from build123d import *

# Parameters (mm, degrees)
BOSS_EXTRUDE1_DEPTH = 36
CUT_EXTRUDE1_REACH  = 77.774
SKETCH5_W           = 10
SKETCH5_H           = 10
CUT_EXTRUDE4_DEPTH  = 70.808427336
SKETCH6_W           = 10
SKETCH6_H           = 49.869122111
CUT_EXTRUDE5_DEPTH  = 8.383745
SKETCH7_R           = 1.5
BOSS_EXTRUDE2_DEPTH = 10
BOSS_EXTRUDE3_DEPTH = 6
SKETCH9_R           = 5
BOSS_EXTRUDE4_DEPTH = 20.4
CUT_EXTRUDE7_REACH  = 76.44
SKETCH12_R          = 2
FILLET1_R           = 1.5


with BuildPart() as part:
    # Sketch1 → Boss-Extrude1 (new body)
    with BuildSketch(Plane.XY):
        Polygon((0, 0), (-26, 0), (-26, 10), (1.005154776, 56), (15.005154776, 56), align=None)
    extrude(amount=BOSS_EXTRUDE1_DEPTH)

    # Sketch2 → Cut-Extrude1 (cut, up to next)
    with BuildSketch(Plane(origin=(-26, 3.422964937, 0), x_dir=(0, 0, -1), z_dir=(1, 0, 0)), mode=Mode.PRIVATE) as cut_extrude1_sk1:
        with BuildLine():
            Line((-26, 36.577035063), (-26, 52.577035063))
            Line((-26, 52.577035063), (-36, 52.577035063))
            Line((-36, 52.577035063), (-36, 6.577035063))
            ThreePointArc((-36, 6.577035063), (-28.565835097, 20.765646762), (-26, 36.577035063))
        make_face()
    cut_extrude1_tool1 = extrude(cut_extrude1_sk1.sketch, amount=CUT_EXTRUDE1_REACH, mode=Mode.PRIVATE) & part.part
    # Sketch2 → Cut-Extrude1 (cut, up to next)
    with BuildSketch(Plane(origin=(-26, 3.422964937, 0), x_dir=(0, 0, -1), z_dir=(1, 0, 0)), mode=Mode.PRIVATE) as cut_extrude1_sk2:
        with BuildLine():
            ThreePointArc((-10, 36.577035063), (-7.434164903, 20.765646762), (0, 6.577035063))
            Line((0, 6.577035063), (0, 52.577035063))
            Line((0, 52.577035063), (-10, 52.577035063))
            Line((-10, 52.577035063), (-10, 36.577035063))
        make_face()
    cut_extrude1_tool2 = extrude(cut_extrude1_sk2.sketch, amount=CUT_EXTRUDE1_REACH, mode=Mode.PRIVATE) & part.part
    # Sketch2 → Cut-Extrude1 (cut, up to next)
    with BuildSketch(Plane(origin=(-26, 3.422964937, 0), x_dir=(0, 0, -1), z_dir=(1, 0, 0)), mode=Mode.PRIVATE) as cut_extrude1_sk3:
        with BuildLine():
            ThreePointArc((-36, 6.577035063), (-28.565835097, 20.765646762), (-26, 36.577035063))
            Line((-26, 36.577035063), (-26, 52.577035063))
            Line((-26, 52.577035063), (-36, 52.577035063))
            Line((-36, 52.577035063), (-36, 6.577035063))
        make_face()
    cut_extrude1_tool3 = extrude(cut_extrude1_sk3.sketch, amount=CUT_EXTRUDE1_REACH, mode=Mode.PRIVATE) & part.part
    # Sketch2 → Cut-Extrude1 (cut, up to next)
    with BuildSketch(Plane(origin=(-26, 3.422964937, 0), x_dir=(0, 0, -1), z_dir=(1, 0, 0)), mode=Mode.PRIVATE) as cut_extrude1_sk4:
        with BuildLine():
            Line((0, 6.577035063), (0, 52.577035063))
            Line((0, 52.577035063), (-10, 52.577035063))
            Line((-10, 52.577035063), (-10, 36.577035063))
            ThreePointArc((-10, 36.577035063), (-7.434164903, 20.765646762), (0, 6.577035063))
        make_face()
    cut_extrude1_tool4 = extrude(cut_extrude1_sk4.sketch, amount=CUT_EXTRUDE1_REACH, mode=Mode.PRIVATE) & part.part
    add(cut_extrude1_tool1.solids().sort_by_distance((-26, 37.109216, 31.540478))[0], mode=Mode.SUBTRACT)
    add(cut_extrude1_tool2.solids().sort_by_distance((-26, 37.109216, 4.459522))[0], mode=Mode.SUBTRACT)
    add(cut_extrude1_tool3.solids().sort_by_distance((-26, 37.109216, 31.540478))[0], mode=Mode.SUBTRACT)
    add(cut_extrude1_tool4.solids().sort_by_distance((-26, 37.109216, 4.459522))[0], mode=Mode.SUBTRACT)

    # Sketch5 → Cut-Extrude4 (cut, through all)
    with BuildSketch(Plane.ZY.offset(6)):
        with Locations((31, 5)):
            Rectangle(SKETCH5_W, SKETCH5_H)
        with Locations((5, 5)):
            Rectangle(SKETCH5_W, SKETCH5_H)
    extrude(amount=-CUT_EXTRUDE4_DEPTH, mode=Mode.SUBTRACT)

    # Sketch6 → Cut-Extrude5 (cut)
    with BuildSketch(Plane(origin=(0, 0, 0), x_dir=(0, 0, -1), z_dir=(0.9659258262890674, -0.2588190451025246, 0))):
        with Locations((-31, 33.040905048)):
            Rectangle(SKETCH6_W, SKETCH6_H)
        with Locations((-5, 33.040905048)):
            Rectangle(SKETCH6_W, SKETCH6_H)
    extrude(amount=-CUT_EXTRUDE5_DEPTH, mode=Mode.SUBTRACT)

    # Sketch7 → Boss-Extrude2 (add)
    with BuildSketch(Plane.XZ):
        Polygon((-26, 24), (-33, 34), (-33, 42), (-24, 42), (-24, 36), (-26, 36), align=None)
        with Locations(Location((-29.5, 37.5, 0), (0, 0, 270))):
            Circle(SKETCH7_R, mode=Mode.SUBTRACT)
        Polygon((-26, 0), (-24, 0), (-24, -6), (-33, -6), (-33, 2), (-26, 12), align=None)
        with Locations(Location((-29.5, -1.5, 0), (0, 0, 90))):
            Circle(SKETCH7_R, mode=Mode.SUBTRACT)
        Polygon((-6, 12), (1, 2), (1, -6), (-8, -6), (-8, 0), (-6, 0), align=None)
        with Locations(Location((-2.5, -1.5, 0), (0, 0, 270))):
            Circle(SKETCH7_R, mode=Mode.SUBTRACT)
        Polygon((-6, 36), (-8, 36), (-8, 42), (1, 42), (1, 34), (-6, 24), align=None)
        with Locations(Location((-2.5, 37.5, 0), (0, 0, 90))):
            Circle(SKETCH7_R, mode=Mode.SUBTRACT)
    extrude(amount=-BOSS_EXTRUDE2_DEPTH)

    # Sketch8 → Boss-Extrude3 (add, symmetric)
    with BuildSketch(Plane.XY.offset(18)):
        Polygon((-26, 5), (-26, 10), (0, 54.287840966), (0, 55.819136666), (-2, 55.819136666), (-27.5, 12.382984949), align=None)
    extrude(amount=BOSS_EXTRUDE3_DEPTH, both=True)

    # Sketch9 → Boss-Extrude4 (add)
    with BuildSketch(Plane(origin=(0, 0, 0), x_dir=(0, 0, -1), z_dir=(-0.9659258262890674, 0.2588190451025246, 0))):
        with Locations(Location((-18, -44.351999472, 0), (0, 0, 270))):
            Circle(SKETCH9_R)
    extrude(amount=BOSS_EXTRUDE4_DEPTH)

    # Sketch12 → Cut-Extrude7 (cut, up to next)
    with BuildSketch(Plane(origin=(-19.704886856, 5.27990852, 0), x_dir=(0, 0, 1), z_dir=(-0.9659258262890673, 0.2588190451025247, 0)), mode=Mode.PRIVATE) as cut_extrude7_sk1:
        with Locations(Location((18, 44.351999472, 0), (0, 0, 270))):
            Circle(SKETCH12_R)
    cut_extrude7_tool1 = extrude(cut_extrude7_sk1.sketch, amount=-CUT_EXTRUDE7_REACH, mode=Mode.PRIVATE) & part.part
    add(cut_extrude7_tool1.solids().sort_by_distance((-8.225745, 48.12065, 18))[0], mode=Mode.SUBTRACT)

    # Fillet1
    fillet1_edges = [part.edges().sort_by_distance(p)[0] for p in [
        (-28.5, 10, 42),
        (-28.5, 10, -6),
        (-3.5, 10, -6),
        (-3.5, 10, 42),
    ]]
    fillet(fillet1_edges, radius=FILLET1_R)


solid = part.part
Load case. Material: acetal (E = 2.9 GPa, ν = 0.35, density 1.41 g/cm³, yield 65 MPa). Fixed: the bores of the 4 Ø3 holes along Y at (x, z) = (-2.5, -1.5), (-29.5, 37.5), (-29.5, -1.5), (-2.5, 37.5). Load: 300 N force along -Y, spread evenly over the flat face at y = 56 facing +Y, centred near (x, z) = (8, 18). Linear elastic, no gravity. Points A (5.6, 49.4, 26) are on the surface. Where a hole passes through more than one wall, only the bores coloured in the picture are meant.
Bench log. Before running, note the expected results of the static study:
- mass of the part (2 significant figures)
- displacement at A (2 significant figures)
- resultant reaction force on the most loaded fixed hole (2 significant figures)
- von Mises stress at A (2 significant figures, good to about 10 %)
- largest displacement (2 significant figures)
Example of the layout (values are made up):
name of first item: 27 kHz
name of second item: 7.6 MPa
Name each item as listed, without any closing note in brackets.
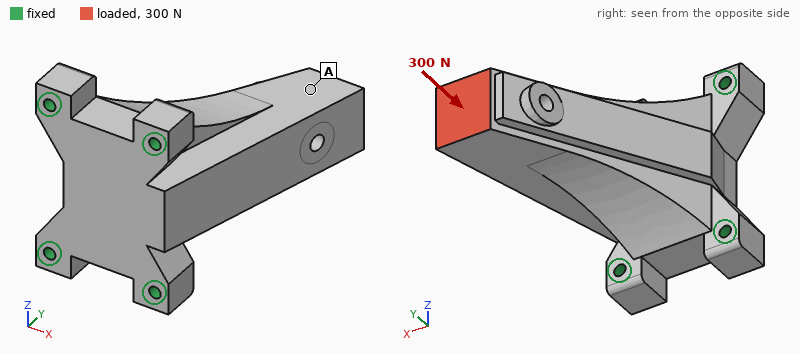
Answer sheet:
mass of the part: 46 g
displacement at A: 0.20 mm
resultant reaction force on the most loaded fixed hole: 220 N
von Mises stress at A: 1.7 MPa
largest displacement: 0.28 mm
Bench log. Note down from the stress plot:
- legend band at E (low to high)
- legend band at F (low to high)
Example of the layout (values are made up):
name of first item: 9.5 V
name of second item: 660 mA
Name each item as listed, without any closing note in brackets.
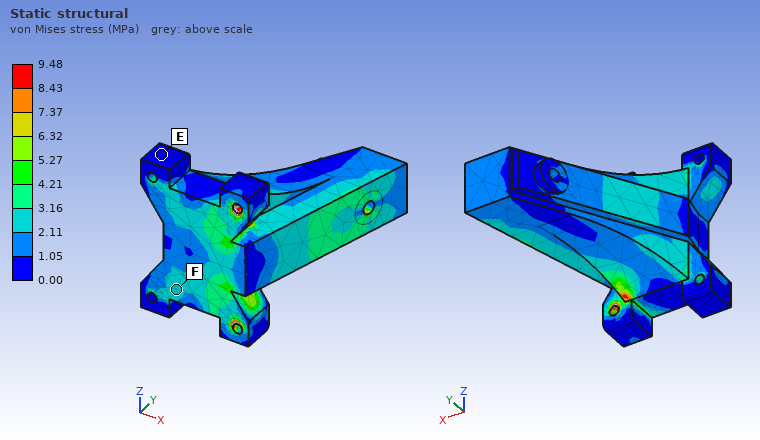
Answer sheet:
legend band at E: 0.00 to 1.05 MPa
legend band at F: 2.11 to 3.16 MPa
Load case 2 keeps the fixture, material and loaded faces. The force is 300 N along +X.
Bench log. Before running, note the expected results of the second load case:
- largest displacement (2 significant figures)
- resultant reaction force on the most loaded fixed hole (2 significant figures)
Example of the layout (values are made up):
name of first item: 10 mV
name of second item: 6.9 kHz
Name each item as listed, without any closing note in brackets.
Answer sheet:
largest displacement: 0.58 mm
resultant reaction force on the most loaded fixed hole: 320 N
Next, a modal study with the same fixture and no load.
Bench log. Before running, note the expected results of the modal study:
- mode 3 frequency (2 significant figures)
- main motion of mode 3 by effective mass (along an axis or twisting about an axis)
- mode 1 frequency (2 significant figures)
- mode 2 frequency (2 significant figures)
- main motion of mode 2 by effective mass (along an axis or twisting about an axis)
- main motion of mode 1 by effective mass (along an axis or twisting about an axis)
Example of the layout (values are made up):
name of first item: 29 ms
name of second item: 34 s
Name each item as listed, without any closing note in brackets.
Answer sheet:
mode 3 frequency: 3800 Hz
main motion of mode 3 by effective mass: along Y
mode 1 frequency: 1400 Hz
mode 2 frequency: 1800 Hz
main motion of mode 2 by effective mass: along Z
main motion of mode 1 by effective mass: along X
